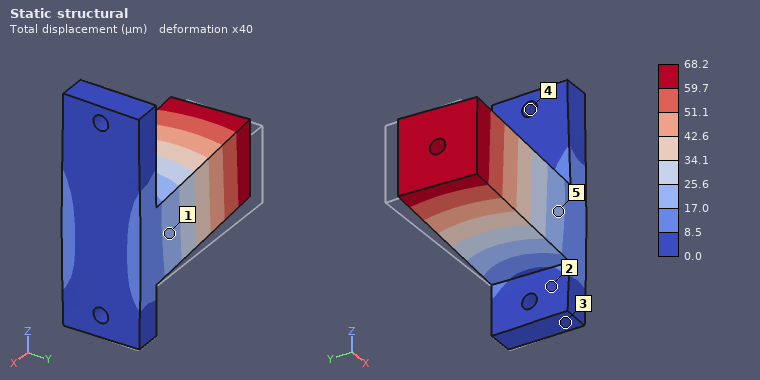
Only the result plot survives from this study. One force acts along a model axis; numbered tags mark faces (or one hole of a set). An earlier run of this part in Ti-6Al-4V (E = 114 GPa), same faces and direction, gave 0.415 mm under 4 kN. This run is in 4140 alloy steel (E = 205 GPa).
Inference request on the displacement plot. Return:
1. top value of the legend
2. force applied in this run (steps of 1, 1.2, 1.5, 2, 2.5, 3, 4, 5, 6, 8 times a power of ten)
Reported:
68.2 µm
1.2 kN
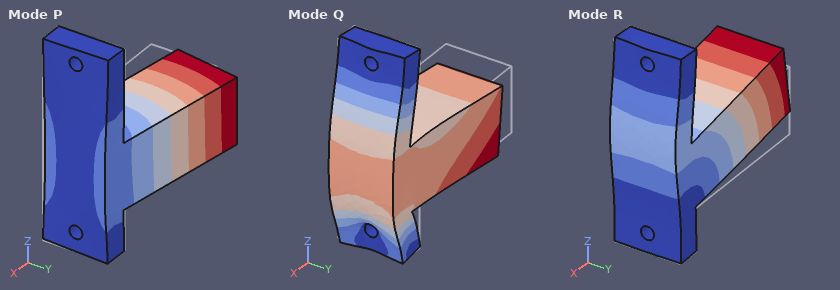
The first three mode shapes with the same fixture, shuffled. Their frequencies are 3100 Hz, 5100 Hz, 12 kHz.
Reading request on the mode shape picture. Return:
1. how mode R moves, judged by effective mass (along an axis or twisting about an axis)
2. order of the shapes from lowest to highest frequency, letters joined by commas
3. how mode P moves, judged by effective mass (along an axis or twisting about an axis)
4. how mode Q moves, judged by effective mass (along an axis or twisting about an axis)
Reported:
along Z
P, R, Q
along Y
along X
